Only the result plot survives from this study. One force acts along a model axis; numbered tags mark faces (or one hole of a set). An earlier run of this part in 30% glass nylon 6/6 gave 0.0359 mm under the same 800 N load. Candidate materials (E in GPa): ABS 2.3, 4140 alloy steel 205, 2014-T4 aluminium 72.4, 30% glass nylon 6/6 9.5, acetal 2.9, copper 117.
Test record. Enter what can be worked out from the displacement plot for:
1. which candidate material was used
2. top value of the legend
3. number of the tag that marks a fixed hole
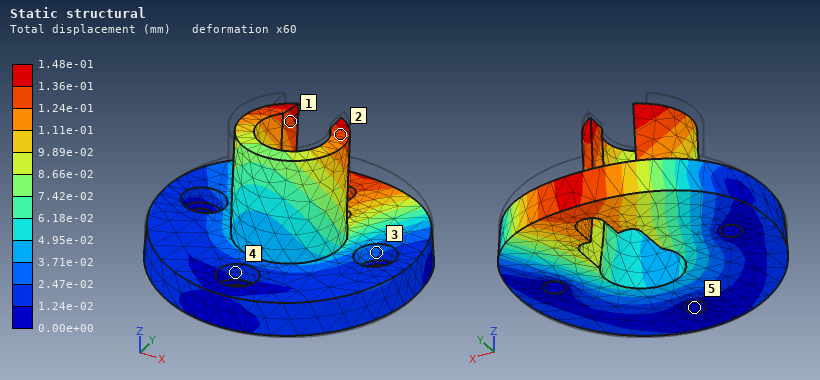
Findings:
ABS
1.48e-01 mm
5
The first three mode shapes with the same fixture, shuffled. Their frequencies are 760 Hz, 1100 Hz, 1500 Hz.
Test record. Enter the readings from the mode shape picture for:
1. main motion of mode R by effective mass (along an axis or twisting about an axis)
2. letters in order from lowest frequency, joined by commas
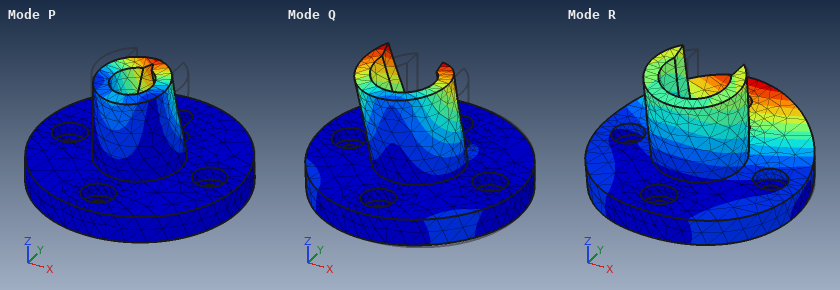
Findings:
along Z
R, Q, P
